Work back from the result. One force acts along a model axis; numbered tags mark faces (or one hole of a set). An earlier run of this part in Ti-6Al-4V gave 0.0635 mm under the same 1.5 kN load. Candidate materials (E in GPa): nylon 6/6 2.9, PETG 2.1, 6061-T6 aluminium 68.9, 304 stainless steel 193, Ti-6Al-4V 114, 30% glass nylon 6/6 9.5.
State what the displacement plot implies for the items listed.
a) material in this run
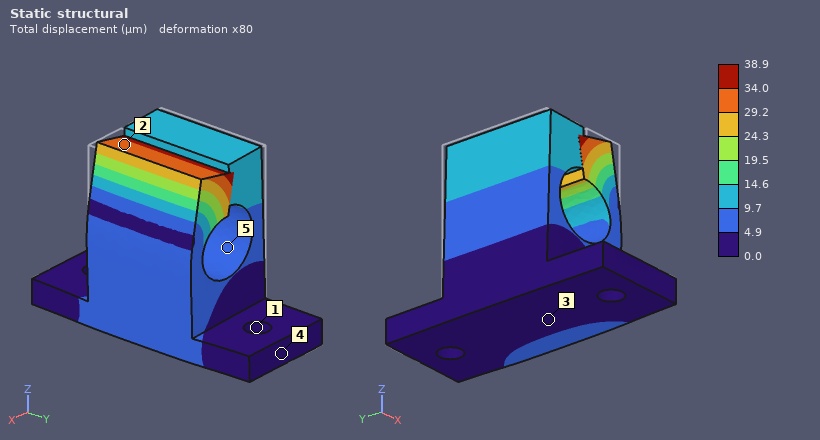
304 stainless steel
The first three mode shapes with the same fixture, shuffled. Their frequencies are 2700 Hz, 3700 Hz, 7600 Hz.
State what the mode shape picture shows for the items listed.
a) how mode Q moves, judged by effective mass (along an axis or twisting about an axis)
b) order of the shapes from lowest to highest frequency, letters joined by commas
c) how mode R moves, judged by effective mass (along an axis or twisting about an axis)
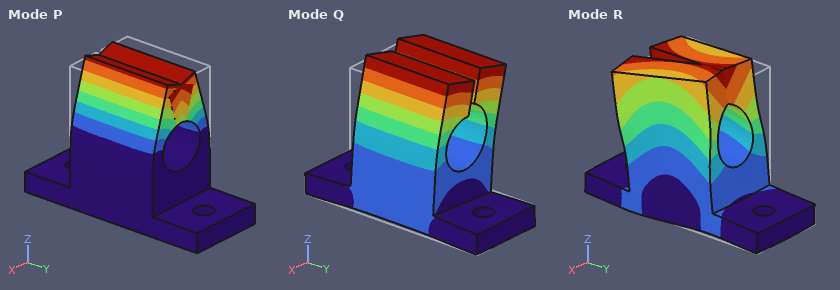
along X
Q, P, R
along Y
